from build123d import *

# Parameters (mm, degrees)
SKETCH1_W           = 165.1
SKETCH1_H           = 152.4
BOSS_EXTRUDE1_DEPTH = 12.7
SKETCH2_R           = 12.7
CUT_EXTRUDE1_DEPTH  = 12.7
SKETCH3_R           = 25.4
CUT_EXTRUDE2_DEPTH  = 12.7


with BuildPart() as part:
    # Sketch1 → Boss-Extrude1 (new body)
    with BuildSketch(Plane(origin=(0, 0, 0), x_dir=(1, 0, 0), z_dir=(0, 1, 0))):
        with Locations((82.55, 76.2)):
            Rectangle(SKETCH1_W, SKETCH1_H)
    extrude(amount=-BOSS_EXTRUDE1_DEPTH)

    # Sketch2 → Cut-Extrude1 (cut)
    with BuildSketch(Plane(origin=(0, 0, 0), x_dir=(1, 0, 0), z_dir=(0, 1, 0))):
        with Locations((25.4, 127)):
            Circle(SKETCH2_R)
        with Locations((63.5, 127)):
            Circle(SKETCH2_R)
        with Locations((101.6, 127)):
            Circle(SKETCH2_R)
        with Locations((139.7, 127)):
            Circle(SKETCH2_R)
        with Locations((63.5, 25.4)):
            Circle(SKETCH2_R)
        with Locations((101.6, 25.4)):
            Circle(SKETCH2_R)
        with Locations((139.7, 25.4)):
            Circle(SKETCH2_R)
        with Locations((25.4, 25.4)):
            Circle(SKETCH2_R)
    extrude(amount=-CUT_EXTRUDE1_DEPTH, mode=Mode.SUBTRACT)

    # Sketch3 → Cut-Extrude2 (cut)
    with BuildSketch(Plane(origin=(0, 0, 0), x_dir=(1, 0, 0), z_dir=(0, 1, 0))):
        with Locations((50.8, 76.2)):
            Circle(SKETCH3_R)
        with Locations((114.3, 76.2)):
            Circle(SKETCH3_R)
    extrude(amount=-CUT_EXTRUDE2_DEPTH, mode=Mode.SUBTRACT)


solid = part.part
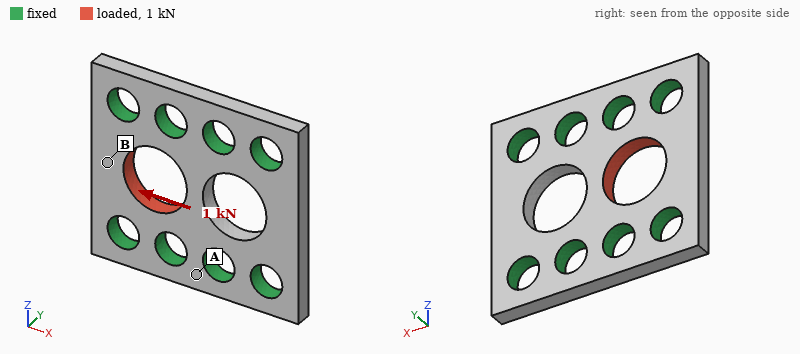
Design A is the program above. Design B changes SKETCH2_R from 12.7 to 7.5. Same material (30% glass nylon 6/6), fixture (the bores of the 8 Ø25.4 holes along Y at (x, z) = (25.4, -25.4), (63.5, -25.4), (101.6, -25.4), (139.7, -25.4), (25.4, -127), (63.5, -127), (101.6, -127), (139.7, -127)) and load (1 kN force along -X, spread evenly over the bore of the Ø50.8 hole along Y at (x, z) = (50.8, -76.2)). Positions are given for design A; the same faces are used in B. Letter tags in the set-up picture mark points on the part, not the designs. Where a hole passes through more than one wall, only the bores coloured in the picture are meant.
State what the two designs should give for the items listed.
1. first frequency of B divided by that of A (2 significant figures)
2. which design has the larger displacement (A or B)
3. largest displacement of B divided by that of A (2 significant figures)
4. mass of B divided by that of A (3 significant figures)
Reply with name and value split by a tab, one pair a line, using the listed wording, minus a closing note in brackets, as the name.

first frequency of B divided by that of A	0.79
which design has the larger displacement	B
largest displacement of B divided by that of A	1.2
mass of B divided by that of A	1.15
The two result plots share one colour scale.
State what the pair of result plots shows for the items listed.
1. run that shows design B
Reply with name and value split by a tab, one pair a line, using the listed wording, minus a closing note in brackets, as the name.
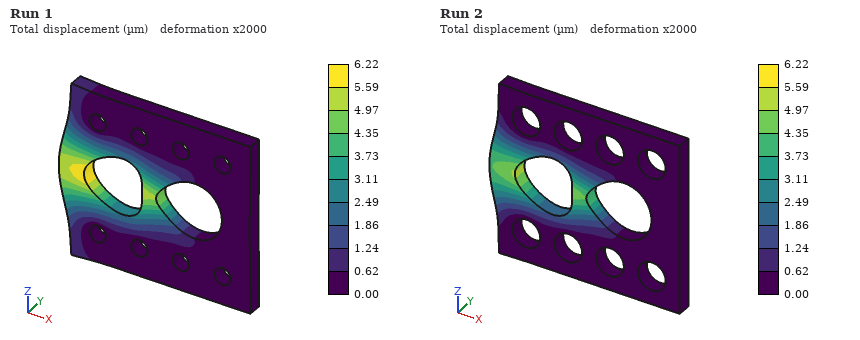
run that shows design B	Run 1
